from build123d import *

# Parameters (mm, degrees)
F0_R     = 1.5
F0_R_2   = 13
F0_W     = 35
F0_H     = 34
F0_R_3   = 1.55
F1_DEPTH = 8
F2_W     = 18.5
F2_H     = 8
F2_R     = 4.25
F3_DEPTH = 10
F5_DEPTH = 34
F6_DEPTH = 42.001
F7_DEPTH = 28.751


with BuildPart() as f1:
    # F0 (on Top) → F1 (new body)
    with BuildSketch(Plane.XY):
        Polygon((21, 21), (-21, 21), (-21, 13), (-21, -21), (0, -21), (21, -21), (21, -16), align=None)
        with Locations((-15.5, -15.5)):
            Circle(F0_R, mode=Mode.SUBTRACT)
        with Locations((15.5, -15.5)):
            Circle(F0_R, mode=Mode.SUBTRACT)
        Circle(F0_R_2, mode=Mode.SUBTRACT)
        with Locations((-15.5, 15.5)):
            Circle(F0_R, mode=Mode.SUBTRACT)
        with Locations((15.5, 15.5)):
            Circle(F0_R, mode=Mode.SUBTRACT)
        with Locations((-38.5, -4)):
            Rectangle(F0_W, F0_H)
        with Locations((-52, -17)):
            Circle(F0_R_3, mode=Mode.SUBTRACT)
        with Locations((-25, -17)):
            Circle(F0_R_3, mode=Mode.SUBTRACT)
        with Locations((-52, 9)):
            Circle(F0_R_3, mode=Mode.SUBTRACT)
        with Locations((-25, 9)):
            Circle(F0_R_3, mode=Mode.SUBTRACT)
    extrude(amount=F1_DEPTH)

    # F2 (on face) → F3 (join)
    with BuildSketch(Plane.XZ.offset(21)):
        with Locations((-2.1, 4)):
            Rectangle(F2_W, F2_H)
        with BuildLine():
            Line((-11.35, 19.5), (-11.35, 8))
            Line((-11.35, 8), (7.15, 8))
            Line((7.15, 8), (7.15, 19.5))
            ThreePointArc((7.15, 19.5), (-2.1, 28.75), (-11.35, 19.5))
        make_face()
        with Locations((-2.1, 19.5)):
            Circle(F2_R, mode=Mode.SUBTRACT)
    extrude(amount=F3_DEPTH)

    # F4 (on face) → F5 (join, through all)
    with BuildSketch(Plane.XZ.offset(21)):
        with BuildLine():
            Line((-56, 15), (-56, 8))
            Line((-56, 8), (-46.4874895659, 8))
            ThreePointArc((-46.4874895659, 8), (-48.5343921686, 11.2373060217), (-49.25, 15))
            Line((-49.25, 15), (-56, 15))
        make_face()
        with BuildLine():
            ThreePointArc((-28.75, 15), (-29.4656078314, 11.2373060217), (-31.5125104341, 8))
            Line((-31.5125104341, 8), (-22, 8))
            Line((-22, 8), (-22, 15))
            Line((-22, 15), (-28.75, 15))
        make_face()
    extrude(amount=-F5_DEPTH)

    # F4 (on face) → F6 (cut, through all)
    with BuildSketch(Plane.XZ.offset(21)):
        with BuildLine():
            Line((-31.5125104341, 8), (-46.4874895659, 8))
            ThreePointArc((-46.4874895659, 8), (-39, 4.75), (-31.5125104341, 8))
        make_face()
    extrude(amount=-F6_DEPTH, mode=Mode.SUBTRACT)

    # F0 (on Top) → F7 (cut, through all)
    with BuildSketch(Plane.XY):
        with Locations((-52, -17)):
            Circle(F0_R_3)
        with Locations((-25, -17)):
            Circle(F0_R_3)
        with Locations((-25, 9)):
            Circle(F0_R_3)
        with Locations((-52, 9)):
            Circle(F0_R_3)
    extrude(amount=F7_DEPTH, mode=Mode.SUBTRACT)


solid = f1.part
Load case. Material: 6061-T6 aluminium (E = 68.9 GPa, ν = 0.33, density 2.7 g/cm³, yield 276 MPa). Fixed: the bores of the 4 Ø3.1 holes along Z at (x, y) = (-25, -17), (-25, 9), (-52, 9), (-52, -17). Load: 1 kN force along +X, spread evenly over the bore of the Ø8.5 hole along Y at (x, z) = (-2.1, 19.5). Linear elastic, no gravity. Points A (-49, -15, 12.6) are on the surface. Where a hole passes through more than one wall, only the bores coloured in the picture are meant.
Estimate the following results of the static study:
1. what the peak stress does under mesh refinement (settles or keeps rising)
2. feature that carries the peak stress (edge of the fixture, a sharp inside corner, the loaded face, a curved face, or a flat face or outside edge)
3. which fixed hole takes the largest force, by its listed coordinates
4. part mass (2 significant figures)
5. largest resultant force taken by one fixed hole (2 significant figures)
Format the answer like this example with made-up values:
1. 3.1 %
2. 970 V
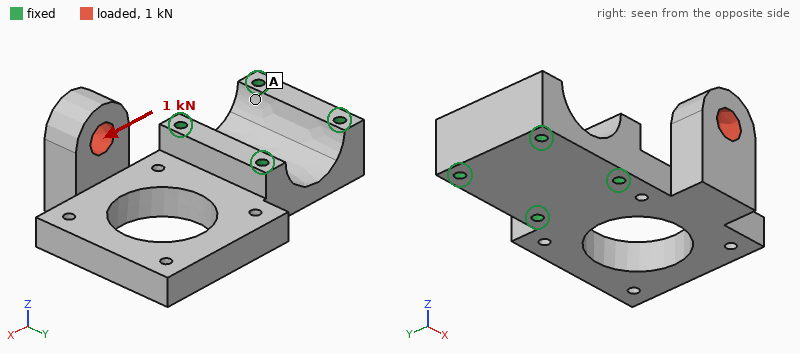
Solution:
1. keeps rising
2. a sharp inside corner
3. (-25, -17)
4. 69 g
5. 1.4 kN
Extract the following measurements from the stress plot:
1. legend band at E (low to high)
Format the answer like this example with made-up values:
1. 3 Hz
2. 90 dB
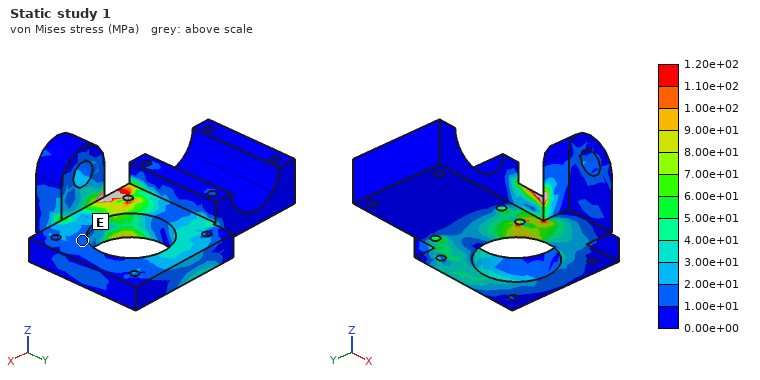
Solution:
1. 1.00e+01 to 2.00e+01 MPa
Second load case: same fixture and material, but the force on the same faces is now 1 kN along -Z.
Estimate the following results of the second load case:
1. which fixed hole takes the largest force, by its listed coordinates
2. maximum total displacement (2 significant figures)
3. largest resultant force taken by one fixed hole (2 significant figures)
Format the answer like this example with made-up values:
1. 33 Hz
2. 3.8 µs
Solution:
1. (-25, -17)
2. 0.24 mm
3. 1.3 kN
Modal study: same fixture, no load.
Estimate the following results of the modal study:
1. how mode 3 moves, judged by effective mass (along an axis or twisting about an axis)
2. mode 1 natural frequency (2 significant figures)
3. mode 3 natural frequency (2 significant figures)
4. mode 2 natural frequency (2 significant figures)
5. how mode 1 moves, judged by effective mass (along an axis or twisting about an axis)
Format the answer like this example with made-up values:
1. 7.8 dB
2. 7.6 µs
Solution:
1. along Y
2. 2300 Hz
3. 5100 Hz
4. 3600 Hz
5. along Z
